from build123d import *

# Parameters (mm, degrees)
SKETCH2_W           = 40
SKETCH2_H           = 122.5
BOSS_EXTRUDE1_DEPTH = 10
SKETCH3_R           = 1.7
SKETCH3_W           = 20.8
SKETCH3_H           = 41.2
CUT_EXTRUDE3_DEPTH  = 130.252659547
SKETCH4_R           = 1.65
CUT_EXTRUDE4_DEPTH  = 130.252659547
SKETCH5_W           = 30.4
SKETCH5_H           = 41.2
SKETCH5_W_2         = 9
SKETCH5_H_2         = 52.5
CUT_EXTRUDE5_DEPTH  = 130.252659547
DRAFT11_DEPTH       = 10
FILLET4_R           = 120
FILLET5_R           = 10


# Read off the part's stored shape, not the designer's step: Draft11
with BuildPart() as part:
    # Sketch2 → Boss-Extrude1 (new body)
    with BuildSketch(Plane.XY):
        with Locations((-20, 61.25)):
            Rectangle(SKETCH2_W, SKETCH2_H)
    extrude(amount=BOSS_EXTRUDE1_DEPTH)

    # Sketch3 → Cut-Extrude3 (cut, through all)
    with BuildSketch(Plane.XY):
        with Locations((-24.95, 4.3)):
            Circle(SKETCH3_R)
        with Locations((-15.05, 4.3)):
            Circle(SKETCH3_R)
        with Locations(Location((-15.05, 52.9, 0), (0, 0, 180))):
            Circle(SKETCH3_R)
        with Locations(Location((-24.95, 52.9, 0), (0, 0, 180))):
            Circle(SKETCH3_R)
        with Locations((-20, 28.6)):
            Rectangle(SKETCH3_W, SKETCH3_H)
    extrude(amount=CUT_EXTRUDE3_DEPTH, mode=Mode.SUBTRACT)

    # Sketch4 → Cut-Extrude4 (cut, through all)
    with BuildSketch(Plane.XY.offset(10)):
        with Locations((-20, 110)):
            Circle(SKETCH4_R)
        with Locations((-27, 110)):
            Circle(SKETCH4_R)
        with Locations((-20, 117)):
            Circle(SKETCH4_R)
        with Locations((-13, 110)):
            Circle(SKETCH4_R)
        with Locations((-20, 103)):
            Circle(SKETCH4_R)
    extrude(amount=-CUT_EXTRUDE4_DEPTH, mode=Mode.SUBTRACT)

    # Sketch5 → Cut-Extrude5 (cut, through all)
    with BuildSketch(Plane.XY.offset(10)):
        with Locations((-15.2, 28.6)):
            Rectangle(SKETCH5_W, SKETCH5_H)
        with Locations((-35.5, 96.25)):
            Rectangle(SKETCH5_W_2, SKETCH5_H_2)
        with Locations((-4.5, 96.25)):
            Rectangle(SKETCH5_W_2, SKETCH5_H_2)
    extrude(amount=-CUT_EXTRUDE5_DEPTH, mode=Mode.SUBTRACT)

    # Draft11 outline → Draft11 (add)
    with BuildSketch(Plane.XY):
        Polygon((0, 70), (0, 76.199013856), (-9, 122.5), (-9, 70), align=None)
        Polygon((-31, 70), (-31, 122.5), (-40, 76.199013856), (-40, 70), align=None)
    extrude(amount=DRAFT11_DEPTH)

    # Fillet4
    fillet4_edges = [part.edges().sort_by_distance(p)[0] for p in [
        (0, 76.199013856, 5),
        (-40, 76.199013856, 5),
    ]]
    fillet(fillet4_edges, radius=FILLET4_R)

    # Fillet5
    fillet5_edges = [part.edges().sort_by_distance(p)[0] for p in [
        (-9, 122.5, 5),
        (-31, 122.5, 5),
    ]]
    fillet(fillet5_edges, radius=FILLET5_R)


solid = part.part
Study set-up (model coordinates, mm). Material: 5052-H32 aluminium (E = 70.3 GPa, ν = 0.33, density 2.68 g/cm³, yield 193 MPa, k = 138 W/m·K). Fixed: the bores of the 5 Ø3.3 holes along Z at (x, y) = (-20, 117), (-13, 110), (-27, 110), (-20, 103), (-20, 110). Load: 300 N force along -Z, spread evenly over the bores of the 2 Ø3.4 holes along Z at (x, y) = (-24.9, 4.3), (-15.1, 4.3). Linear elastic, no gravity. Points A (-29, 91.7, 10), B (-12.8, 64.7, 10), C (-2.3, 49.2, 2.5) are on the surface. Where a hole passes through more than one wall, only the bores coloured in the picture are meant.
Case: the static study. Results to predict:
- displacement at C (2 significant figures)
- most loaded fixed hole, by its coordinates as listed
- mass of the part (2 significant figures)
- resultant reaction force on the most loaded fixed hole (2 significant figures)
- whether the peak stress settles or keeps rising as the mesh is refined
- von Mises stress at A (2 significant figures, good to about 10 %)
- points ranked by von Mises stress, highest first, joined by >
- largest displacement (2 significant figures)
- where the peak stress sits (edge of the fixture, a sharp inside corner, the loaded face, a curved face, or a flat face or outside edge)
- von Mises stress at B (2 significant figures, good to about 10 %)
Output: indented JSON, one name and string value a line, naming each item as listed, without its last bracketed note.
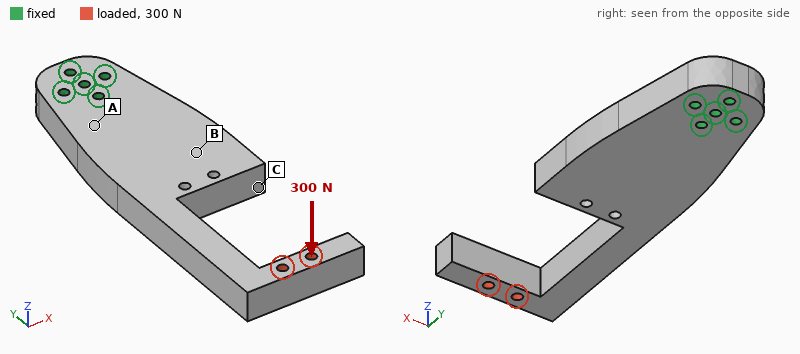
{
  "displacement at C": "0.18 mm",
  "most loaded fixed hole, by its coordinates as listed": "(-20, 103)",
  "mass of the part": "84 g",
  "resultant reaction force on the most loaded fixed hole": "1.4 kN",
  "whether the peak stress settles or keeps rising as the mesh is refined": "keeps rising",
  "von Mises stress at A": "45 MPa",
  "points ranked by von Mises stress, highest first, joined by >": "A > B > C",
  "largest displacement": "1.0 mm",
  "where the peak stress sits": "edge of the fixture",
  "von Mises stress at B": "23 MPa"
}
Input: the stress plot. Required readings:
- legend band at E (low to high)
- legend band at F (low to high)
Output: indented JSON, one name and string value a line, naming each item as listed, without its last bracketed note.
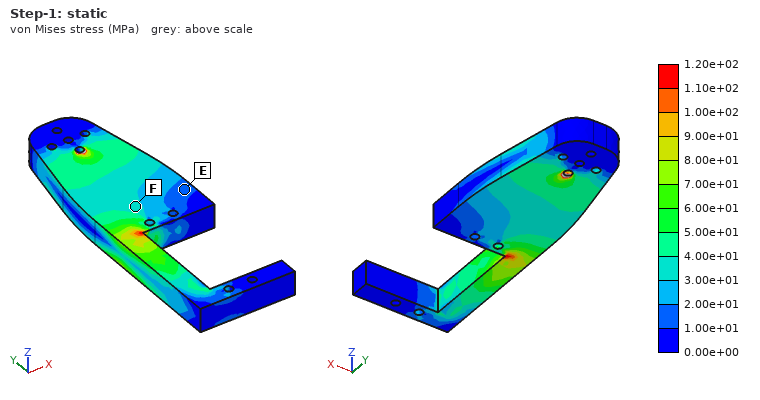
{
  "legend band at E": "1.00e+01 to 2.00e+01 MPa",
  "legend band at F": "3.00e+01 to 4.00e+01 MPa"
}
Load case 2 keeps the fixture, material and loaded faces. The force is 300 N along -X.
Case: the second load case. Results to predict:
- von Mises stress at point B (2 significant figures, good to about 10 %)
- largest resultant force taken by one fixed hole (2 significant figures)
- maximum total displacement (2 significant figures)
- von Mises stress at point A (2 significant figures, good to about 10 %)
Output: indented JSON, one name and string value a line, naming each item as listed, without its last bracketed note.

{
  "von Mises stress at point B": "6.1 MPa",
  "largest resultant force taken by one fixed hole": "1.3 kN",
  "maximum total displacement": "0.44 mm",
  "von Mises stress at point A": "8.0 MPa"
}
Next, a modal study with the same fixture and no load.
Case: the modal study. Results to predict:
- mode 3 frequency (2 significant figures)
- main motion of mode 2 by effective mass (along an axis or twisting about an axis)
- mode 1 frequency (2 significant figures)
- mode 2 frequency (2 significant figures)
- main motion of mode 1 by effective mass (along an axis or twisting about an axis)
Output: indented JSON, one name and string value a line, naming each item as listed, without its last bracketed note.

{
  "mode 3 frequency": "2500 Hz",
  "main motion of mode 2 by effective mass": "along X",
  "mode 1 frequency": "860 Hz",
  "mode 2 frequency": "1400 Hz",
  "main motion of mode 1 by effective mass": "along Z"
}
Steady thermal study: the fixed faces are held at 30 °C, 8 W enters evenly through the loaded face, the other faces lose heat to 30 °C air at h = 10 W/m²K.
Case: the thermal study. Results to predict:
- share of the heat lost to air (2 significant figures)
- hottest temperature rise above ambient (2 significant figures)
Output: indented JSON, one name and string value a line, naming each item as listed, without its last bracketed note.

{
  "share of the heat lost to air": "15 %",
  "hottest temperature rise above ambient": "46 K"
}
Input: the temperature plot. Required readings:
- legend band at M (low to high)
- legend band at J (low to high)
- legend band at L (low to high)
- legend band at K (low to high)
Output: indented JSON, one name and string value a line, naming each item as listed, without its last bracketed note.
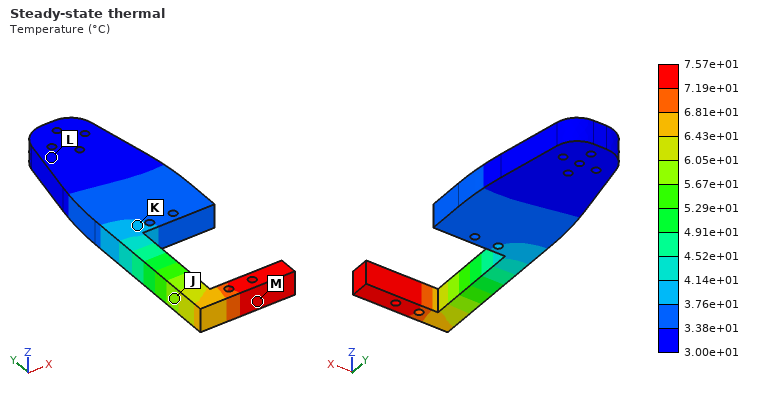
{
  "legend band at M": "7.19e+01 to 7.57e+01 °C",
  "legend band at J": "5.67e+01 to 6.05e+01 °C",
  "legend band at L": "3.00e+01 to 3.38e+01 °C",
  "legend band at K": "3.76e+01 to 4.14e+01 °C"
}
